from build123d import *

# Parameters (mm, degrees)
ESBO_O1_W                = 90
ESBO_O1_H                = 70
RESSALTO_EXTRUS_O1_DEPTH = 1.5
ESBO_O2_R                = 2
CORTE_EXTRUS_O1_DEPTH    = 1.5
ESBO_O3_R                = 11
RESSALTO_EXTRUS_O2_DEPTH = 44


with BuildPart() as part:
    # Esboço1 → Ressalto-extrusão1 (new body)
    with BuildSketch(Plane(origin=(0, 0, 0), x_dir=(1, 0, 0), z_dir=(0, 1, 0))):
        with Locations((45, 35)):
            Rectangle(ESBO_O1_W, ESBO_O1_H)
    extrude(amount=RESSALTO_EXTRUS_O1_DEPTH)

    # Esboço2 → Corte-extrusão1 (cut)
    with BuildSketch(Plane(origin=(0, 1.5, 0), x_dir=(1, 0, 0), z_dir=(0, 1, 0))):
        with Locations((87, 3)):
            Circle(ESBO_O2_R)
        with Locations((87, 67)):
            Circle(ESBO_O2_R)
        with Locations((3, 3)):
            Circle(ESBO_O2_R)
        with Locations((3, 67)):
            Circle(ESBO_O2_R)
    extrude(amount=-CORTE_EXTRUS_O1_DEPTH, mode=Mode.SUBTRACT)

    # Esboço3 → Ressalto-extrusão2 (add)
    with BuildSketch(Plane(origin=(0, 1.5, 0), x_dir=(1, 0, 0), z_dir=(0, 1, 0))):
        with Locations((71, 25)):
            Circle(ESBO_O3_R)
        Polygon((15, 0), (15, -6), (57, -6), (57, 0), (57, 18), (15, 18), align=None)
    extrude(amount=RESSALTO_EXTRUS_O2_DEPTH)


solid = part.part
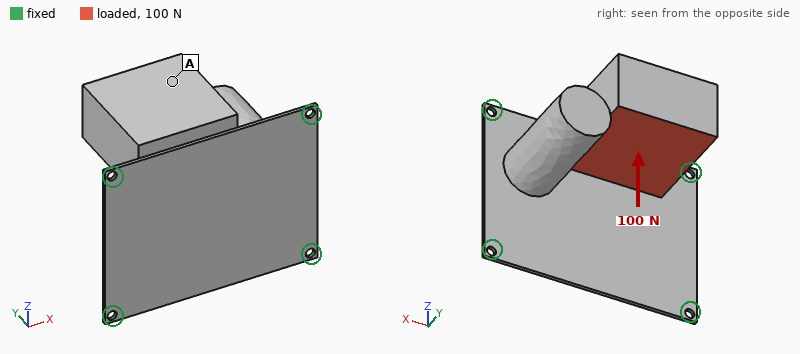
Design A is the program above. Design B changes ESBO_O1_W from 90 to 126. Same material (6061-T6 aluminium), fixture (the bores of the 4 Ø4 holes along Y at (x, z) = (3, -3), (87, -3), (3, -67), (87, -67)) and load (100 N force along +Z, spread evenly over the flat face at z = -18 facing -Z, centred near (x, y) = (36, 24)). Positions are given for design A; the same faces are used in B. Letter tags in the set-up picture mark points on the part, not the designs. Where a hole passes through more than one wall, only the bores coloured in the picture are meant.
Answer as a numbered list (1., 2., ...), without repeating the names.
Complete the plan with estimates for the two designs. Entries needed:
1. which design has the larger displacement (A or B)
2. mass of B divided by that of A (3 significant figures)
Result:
1. A
2. 1.05
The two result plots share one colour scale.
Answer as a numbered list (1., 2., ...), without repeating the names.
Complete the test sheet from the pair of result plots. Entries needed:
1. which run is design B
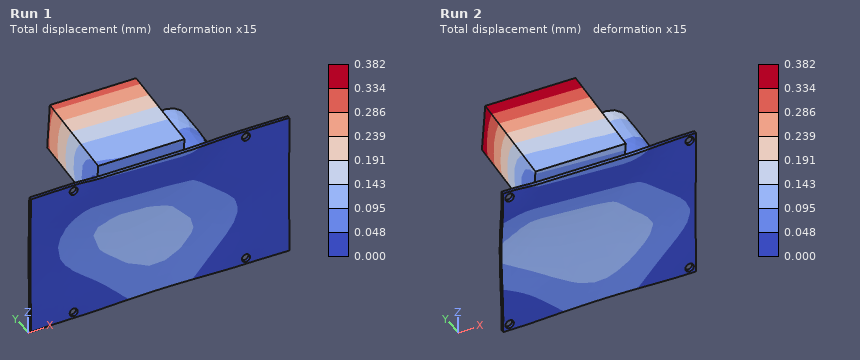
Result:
1. Run 1
